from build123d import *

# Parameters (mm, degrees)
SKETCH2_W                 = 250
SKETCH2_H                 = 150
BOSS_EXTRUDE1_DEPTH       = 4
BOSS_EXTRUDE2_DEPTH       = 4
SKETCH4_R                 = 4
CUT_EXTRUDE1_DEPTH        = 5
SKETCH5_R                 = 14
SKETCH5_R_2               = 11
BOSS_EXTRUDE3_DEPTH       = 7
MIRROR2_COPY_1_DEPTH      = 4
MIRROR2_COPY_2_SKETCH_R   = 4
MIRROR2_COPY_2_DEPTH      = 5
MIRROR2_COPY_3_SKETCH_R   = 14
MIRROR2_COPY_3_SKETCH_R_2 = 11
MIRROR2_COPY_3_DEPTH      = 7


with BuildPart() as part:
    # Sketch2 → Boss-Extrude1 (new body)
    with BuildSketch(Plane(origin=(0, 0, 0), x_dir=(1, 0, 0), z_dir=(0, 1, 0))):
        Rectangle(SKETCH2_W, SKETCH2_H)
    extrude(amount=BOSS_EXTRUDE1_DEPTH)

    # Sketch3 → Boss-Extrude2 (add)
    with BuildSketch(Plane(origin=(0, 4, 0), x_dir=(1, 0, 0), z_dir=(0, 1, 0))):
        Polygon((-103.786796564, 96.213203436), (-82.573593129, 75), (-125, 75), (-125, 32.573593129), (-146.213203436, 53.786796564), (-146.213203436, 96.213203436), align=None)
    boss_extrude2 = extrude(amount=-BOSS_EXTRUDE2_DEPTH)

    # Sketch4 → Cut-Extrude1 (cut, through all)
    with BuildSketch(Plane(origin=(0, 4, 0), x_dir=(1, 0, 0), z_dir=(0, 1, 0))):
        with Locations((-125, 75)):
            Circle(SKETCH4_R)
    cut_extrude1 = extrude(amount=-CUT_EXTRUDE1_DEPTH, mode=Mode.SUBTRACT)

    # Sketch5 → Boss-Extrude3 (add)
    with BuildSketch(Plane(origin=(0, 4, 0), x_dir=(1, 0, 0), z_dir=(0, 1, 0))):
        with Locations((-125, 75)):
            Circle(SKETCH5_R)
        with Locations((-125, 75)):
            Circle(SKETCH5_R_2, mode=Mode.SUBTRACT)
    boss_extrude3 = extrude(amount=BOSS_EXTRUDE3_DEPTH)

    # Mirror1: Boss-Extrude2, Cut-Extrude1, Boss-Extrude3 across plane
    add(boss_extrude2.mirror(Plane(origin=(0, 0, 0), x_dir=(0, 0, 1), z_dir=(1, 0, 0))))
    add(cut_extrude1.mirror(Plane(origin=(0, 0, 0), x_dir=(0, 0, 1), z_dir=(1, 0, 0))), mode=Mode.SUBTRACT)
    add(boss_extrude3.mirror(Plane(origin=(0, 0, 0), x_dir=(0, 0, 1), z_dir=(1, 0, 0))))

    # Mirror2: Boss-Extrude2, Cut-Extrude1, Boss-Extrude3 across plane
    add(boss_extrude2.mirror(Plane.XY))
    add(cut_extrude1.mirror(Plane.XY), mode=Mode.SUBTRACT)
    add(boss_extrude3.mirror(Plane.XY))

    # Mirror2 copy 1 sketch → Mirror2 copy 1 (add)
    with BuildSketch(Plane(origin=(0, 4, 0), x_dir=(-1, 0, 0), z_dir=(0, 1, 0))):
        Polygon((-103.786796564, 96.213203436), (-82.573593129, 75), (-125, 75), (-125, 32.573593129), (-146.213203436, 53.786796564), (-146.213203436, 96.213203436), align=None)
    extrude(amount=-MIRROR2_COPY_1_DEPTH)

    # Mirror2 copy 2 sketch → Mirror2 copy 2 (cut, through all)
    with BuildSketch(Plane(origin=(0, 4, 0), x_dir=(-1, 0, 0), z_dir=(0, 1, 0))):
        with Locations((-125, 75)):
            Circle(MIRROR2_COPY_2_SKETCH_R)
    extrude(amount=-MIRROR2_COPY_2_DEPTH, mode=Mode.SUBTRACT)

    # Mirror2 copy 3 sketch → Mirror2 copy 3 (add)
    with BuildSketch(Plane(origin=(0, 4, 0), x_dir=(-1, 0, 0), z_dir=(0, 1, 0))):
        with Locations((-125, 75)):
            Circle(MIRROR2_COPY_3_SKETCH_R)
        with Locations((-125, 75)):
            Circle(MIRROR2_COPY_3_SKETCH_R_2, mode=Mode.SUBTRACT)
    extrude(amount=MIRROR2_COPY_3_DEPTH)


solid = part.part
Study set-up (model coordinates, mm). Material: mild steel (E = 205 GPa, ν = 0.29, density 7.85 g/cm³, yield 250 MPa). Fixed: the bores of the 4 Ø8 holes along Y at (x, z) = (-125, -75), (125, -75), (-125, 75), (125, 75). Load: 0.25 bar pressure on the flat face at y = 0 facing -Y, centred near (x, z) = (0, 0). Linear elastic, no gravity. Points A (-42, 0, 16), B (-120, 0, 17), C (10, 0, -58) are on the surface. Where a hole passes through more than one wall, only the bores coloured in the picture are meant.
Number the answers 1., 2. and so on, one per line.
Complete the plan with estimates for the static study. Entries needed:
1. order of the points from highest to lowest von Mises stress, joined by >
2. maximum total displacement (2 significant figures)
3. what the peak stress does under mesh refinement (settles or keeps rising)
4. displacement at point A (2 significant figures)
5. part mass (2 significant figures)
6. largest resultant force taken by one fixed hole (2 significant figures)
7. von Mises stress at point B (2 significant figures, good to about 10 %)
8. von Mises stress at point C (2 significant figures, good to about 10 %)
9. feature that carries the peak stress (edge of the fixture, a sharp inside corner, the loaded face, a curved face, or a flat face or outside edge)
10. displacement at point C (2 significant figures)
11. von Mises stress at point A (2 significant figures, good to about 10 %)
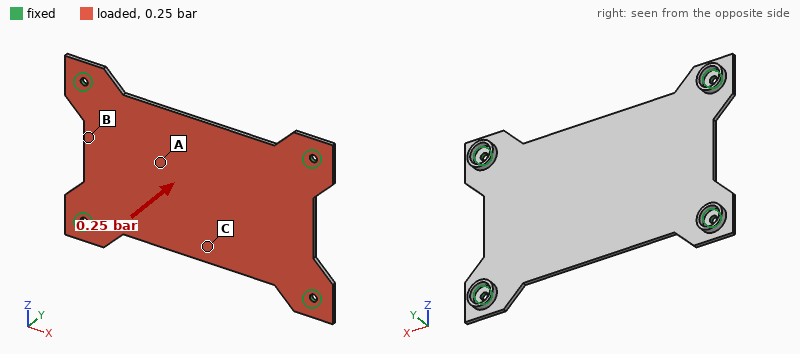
1. C > A > B
2. 0.29 mm
3. keeps rising
4. 0.24 mm
5. 1.4 kg
6. 280 N
7. 11 MPa
8. 26 MPa
9. edge of the fixture
10. 0.27 mm
11. 17 MPa
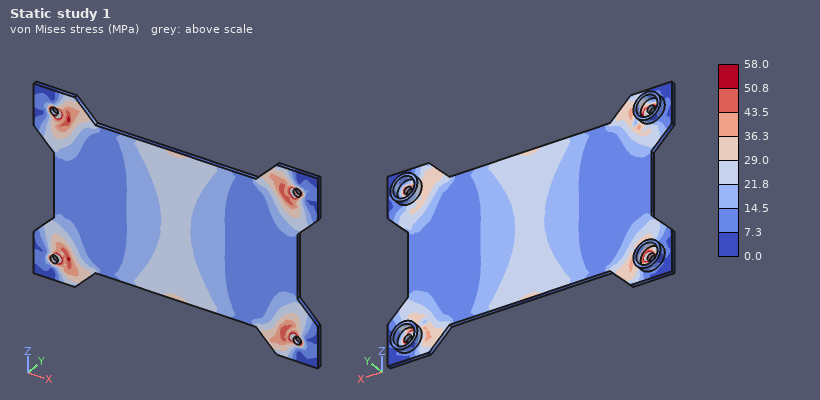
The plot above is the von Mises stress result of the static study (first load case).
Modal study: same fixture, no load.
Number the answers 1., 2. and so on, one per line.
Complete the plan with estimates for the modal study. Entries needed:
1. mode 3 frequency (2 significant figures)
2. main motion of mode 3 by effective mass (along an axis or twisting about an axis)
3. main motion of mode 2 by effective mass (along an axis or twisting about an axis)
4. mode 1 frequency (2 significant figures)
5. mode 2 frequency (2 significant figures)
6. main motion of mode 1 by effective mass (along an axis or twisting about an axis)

1. 770 Hz
2. twisting about Z
3. twisting about X
4. 310 Hz
5. 560 Hz
6. along Y
